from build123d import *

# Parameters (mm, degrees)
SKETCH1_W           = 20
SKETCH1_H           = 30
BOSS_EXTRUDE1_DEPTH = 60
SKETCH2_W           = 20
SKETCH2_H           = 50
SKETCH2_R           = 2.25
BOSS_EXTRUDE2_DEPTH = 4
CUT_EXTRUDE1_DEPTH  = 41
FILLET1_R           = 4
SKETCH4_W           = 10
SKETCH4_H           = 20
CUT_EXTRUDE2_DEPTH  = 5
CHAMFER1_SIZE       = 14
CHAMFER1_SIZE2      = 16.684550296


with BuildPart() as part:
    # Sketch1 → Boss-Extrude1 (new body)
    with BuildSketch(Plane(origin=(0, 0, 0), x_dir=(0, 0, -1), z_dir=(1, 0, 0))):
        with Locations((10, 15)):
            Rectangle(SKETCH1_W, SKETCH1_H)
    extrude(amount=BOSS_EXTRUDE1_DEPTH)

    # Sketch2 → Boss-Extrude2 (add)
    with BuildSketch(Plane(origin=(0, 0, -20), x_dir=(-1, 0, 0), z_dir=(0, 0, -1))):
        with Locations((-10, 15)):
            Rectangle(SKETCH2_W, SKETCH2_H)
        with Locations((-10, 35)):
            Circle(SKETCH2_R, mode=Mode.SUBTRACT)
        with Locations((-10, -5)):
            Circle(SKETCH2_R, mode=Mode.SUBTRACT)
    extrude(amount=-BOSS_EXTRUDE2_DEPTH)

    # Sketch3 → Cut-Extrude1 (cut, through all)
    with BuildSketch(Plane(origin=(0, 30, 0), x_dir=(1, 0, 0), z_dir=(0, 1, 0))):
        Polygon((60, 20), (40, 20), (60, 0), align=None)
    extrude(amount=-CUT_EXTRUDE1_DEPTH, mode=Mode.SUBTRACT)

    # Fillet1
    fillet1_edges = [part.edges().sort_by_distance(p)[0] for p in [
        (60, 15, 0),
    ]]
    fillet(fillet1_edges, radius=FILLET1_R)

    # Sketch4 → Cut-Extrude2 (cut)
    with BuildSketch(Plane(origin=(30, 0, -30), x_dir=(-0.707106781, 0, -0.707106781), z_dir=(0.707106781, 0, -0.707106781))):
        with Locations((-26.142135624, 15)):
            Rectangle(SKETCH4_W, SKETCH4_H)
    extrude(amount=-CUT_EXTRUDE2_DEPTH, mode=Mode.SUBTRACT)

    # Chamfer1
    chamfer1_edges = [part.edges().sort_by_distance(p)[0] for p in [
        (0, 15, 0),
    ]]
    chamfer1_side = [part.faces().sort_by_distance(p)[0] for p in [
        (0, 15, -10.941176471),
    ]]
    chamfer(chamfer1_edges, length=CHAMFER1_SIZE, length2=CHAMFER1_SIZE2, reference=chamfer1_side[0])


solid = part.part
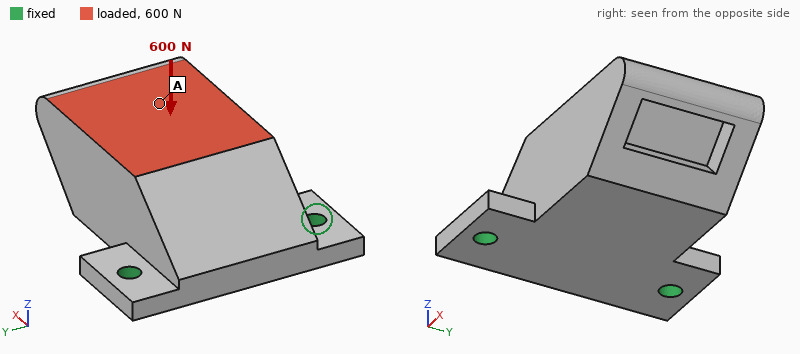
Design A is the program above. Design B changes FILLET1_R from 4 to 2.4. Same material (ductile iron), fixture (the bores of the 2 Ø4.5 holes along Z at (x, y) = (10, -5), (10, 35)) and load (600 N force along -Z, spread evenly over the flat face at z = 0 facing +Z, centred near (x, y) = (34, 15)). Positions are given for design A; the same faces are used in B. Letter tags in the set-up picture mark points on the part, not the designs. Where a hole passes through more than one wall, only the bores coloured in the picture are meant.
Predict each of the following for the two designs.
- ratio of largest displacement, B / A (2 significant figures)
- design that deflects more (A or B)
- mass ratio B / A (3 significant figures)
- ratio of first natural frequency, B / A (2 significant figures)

1.1
B
1.01
0.97
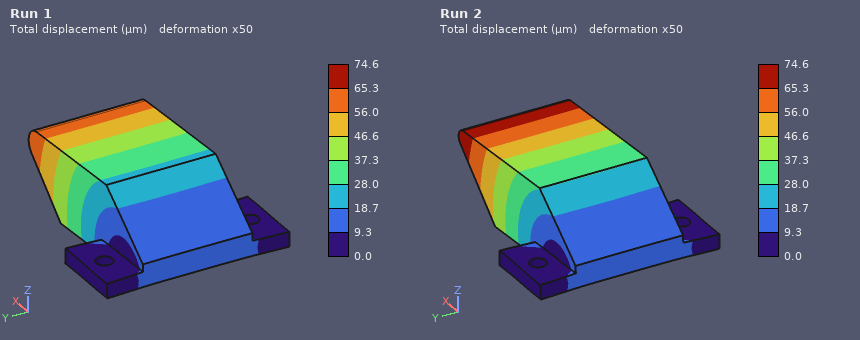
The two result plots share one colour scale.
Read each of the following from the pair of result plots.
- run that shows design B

Run 2
